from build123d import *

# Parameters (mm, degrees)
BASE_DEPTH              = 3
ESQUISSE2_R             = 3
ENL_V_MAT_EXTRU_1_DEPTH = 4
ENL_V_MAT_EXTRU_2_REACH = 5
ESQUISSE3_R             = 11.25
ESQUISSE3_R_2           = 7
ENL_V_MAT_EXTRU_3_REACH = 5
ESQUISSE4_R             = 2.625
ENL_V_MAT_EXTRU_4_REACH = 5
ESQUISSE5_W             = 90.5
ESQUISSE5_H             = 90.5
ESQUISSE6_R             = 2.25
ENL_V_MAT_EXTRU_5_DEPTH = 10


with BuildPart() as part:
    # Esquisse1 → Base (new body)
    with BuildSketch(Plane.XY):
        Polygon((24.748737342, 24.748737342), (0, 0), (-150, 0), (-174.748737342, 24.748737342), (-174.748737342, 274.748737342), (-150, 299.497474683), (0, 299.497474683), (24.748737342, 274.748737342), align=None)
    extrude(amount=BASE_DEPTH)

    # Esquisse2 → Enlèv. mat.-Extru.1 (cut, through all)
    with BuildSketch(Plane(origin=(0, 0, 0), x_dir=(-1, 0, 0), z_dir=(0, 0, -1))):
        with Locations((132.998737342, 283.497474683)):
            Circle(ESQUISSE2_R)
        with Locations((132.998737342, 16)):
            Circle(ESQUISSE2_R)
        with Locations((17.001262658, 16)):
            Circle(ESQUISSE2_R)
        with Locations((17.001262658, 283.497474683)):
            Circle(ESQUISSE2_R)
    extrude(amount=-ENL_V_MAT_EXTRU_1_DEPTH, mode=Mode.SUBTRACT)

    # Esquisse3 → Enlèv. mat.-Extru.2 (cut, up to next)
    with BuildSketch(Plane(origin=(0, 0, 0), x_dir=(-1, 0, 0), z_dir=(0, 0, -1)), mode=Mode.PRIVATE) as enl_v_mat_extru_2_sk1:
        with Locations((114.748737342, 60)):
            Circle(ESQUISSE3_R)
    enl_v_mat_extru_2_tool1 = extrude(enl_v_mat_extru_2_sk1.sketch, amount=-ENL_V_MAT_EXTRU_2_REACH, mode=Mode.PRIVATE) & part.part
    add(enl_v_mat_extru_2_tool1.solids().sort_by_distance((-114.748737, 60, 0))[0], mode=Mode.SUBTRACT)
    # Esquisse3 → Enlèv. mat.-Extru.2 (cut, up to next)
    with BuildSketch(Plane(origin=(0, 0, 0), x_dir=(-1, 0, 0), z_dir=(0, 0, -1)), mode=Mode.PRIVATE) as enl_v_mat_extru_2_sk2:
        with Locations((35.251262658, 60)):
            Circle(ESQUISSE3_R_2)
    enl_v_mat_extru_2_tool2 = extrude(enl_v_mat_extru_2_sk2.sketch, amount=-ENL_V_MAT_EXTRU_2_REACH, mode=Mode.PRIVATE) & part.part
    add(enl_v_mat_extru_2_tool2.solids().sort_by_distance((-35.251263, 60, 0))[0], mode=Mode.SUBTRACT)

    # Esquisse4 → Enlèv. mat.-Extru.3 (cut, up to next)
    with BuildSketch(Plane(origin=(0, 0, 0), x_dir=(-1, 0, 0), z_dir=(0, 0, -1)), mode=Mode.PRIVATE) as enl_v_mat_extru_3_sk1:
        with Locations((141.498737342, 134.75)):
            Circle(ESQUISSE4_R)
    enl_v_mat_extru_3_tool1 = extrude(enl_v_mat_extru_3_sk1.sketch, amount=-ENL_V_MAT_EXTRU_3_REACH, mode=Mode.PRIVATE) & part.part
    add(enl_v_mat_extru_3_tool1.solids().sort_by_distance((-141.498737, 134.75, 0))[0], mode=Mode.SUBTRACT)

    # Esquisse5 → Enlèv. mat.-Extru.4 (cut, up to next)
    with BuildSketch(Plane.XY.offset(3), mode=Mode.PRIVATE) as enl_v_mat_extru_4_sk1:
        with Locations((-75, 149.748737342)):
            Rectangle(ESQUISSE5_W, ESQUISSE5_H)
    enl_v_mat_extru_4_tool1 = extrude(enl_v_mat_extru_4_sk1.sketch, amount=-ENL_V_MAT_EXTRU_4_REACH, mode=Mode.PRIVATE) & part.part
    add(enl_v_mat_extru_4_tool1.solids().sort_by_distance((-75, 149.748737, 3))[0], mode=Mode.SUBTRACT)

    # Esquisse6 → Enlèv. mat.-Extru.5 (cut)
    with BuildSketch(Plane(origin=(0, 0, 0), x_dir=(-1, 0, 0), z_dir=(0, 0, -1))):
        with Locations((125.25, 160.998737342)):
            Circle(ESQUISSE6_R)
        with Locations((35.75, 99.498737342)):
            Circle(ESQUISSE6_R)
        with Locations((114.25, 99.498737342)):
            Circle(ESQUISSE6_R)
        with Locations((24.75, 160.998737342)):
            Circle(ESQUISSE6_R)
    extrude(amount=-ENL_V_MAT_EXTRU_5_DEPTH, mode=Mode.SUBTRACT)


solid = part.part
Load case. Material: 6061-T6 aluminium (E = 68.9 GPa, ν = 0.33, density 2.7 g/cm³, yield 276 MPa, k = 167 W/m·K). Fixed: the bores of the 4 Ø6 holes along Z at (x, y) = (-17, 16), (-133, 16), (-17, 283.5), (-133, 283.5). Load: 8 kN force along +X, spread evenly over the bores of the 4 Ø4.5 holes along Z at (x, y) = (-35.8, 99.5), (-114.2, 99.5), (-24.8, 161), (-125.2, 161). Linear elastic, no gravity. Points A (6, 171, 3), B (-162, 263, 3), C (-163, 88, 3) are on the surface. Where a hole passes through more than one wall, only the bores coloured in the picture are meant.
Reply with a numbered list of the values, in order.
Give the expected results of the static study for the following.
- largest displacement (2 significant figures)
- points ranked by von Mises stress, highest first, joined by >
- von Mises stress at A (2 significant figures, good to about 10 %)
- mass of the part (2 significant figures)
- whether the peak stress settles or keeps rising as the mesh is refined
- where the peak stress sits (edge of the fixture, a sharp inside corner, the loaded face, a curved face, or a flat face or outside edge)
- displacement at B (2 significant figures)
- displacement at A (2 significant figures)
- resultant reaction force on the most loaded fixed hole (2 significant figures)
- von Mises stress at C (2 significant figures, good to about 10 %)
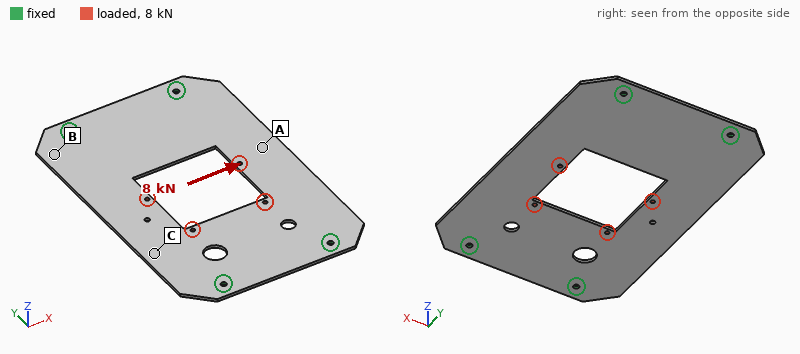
1. 81 µm
2. A > C > B
3. 23 MPa
4. 400 g
5. keeps rising
6. edge of the fixture
7. 15 µm
8. 60 µm
9. 2.9 kN
10. 12 MPa
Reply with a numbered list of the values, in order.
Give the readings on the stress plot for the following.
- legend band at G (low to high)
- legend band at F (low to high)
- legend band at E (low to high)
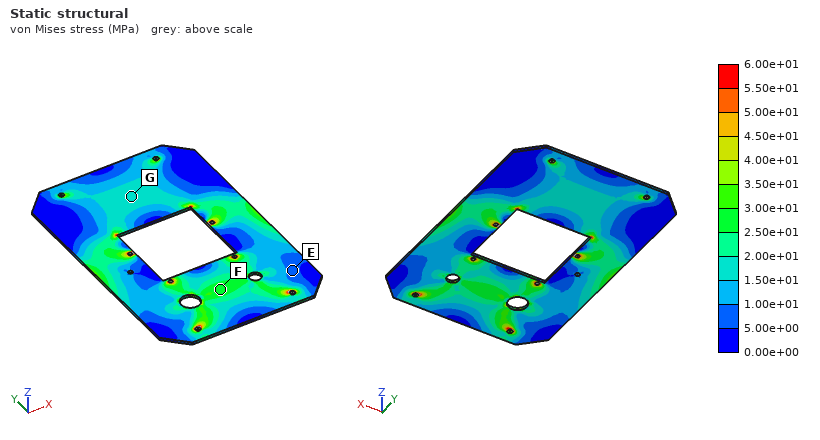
1. 1.50e+01 to 2.00e+01 MPa
2. 2.50e+01 to 3.00e+01 MPa
3. 5.00e+00 to 1.00e+01 MPa
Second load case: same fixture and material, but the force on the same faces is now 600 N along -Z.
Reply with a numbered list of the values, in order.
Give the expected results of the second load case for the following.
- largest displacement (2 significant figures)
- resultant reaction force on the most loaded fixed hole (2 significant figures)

1. 3.0 mm
2. 180 N
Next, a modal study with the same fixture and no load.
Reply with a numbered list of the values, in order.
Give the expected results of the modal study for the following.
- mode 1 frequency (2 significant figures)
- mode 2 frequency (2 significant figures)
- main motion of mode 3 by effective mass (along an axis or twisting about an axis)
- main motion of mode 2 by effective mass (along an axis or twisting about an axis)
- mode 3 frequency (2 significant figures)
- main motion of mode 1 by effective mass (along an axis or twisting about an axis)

1. 210 Hz
2. 260 Hz
3. twisting about X
4. twisting about Y
5. 480 Hz
6. along Z
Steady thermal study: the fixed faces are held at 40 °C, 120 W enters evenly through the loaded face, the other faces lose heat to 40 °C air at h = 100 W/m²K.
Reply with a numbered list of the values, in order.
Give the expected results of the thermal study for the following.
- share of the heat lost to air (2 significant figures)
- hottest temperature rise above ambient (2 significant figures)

1. 88 %
2. 59 K
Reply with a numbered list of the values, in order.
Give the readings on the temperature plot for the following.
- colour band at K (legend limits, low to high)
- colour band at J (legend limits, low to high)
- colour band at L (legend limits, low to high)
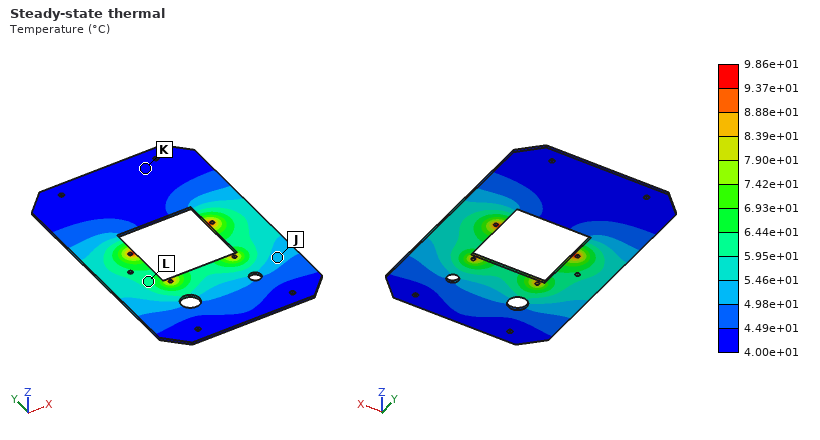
1. 4.00e+01 to 4.49e+01 °C
2. 4.98e+01 to 5.46e+01 °C
3. 5.95e+01 to 6.44e+01 °C
